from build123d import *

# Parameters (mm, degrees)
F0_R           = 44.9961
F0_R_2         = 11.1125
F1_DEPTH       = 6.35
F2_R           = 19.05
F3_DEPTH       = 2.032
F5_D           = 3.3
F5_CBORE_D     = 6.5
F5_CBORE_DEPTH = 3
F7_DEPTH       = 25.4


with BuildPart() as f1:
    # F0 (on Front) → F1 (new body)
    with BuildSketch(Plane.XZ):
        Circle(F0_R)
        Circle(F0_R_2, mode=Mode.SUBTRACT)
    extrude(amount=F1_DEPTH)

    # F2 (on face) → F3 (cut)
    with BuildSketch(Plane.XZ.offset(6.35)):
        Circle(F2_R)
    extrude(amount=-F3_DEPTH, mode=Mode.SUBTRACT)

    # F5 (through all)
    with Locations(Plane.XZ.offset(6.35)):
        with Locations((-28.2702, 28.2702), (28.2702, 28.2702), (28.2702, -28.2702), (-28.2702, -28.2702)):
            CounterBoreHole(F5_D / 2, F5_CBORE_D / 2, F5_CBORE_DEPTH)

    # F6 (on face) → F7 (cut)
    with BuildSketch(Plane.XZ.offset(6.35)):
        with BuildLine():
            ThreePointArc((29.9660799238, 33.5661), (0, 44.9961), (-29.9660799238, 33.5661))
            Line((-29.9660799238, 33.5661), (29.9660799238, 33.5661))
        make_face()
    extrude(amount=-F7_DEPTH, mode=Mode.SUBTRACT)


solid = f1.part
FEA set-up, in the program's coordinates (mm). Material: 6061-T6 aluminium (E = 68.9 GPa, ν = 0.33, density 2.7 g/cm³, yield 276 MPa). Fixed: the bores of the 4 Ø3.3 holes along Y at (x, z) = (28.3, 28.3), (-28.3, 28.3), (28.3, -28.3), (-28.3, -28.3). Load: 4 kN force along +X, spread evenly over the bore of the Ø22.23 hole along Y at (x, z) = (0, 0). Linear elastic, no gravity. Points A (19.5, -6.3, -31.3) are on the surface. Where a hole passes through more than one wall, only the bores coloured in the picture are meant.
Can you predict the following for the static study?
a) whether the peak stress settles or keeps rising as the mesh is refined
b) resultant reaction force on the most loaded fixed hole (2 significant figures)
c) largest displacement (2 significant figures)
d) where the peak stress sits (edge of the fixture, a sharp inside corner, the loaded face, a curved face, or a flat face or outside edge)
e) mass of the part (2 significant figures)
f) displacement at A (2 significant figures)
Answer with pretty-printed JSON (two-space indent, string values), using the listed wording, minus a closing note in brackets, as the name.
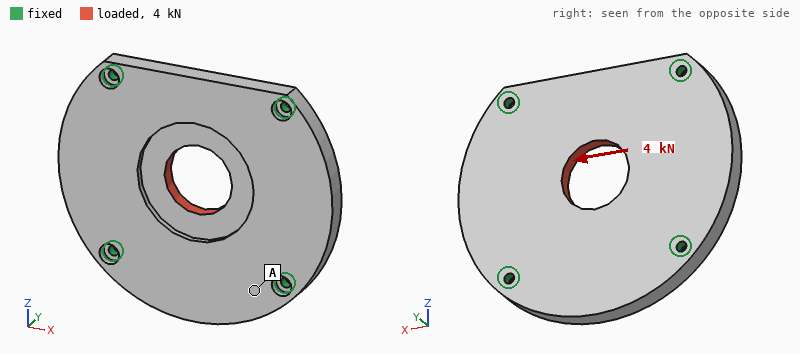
{
  "whether the peak stress settles or keeps rising as the mesh is refined": "keeps rising",
  "resultant reaction force on the most loaded fixed hole": "1.0 kN",
  "largest displacement": "8.0 µm",
  "where the peak stress sits": "edge of the fixture",
  "mass of the part": "89 g",
  "displacement at A": "2.5 µm"
}
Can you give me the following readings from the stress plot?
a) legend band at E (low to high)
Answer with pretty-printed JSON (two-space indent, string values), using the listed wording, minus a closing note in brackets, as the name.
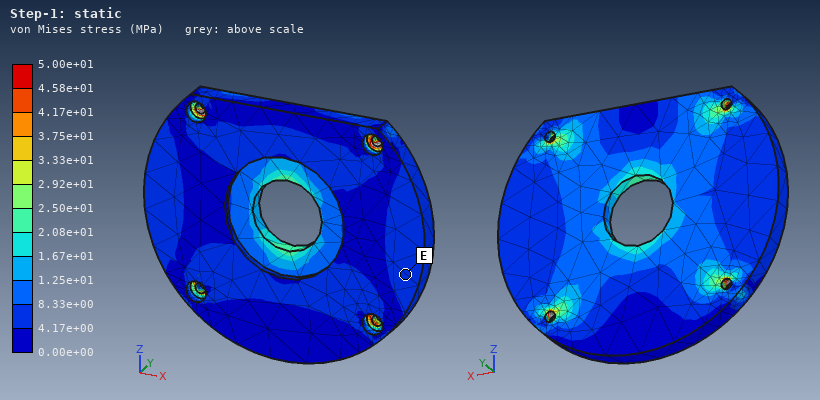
{
  "legend band at E": "4.17e+00 to 8.33e+00 MPa"
}
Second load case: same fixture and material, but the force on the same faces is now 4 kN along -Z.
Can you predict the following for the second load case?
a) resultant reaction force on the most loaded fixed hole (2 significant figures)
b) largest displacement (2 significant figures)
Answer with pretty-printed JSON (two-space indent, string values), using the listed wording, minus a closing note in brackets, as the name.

{
  "resultant reaction force on the most loaded fixed hole": "1.1 kN",
  "largest displacement": "9.5 µm"
}
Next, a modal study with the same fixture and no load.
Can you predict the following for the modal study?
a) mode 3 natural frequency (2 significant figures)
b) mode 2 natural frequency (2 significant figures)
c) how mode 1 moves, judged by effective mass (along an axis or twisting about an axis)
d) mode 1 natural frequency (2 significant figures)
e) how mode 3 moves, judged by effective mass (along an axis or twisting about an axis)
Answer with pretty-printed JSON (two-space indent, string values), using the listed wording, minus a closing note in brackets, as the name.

{
  "mode 3 natural frequency": "6500 Hz",
  "mode 2 natural frequency": "5700 Hz",
  "how mode 1 moves, judged by effective mass": "along Y",
  "mode 1 natural frequency": "5300 Hz",
  "how mode 3 moves, judged by effective mass": "twisting about Z"
}
